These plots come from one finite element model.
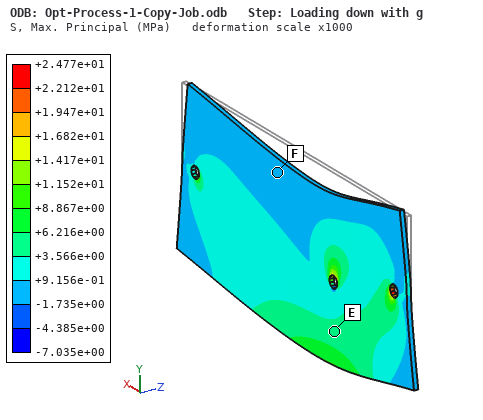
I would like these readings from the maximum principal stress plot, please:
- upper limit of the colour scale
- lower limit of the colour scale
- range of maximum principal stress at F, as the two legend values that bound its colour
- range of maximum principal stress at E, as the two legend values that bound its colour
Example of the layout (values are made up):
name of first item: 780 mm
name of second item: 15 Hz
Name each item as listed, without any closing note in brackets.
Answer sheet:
upper limit of the colour scale: +2.477e+01 MPa
lower limit of the colour scale: -7.035e+00 MPa
range of maximum principal stress at F, as the two legend values that bound its colour: -1.735e+00 to +9.156e-01 MPa
range of maximum principal stress at E, as the two legend values that bound its colour: +3.566e+00 to +6.216e+00 MPa
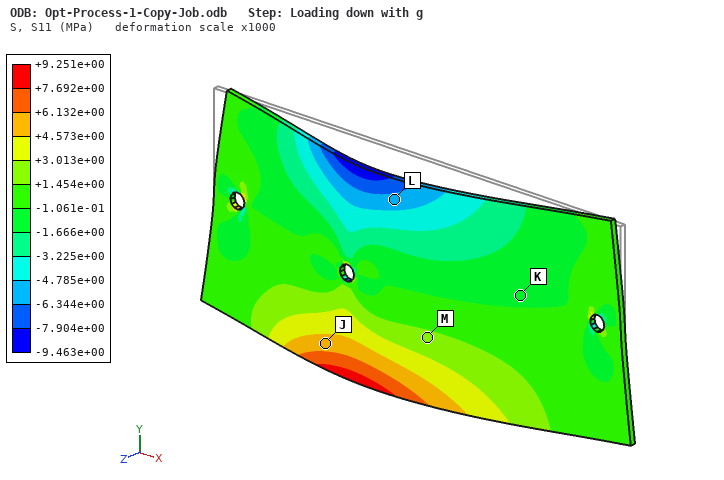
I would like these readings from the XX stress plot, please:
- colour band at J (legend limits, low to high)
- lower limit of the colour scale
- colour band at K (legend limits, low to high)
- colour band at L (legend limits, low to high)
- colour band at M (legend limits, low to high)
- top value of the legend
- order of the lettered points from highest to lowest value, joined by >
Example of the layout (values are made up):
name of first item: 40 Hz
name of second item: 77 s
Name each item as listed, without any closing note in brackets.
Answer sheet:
colour band at J: +4.573e+00 to +6.132e+00 MPa
lower limit of the colour scale: -9.463e+00 MPa
colour band at K: -1.666e+00 to -1.061e-01 MPa
colour band at L: -6.344e+00 to -4.785e+00 MPa
colour band at M: +1.454e+00 to +3.013e+00 MPa
top value of the legend: +9.251e+00 MPa
order of the lettered points from highest to lowest value, joined by >: J > M > K > L
